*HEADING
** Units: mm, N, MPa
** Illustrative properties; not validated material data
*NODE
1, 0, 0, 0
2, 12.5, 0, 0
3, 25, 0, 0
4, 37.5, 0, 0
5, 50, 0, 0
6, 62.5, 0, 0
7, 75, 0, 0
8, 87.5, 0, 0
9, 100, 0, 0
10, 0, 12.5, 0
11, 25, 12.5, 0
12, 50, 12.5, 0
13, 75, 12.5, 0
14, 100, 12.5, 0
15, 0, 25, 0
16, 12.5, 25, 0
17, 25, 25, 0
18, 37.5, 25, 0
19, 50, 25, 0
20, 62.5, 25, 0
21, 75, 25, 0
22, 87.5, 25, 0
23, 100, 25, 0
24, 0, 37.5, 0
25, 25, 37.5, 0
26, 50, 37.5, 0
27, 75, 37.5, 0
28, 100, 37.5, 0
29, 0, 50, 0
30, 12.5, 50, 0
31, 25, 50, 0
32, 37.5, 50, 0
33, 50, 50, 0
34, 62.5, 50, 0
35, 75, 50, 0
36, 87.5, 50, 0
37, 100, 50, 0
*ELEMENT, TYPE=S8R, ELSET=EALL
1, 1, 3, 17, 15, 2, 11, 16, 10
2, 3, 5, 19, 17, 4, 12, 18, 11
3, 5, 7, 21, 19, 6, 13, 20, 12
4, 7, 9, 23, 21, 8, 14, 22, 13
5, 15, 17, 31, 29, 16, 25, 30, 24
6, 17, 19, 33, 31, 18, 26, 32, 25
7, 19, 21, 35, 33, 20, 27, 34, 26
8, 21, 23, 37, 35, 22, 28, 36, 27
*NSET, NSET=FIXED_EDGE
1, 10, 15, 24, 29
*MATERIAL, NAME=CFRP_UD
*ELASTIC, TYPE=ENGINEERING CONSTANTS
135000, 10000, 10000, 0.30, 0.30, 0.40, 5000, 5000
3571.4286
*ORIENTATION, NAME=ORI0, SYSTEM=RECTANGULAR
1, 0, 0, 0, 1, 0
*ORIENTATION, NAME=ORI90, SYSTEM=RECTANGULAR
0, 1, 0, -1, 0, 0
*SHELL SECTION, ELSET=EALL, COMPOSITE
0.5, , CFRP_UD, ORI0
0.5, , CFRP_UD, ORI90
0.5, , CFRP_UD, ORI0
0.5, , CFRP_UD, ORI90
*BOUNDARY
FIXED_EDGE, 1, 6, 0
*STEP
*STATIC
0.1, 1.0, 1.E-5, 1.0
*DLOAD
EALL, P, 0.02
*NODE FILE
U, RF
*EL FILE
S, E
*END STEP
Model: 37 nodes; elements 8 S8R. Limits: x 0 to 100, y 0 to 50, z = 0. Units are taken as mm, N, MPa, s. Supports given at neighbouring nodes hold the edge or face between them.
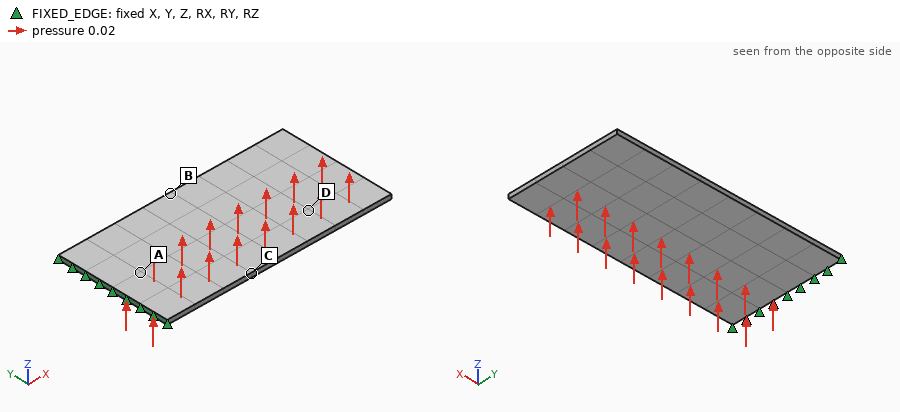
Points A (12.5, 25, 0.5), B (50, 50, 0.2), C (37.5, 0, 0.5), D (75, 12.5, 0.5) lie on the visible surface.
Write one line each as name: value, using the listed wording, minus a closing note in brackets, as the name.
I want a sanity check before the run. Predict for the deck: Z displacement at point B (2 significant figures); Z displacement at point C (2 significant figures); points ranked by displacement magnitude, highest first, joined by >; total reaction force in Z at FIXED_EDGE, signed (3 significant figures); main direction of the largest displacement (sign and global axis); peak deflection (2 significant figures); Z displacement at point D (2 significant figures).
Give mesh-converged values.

Z displacement at point B: 2.1 mm
Z displacement at point C: 1.3 mm
points ranked by displacement magnitude, highest first, joined by >: D > B > C > A
total reaction force in Z at FIXED_EDGE, signed: -100 N
main direction of the largest displacement: +Z
peak deflection: 6.0 mm
Z displacement at point D: 4.0 mm
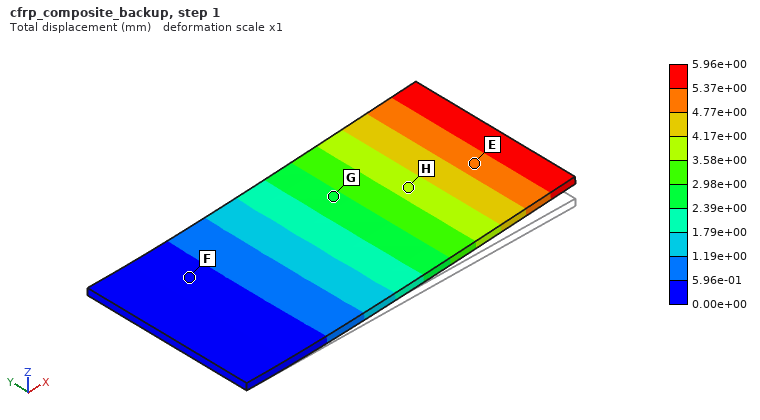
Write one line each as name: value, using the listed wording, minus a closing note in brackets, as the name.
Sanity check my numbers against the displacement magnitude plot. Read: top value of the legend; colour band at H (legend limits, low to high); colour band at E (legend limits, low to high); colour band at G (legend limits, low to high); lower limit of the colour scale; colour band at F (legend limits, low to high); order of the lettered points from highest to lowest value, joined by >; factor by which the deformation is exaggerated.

top value of the legend: 5.96e+00 mm
colour band at H: 3.58e+00 to 4.17e+00 mm
colour band at E: 4.77e+00 to 5.37e+00 mm
colour band at G: 2.39e+00 to 2.98e+00 mm
lower limit of the colour scale: 0.00e+00 mm
colour band at F: 0.00e+00 to 5.96e-01 mm
order of the lettered points from highest to lowest value, joined by >: E > H > G > F
factor by which the deformation is exaggerated: 1
